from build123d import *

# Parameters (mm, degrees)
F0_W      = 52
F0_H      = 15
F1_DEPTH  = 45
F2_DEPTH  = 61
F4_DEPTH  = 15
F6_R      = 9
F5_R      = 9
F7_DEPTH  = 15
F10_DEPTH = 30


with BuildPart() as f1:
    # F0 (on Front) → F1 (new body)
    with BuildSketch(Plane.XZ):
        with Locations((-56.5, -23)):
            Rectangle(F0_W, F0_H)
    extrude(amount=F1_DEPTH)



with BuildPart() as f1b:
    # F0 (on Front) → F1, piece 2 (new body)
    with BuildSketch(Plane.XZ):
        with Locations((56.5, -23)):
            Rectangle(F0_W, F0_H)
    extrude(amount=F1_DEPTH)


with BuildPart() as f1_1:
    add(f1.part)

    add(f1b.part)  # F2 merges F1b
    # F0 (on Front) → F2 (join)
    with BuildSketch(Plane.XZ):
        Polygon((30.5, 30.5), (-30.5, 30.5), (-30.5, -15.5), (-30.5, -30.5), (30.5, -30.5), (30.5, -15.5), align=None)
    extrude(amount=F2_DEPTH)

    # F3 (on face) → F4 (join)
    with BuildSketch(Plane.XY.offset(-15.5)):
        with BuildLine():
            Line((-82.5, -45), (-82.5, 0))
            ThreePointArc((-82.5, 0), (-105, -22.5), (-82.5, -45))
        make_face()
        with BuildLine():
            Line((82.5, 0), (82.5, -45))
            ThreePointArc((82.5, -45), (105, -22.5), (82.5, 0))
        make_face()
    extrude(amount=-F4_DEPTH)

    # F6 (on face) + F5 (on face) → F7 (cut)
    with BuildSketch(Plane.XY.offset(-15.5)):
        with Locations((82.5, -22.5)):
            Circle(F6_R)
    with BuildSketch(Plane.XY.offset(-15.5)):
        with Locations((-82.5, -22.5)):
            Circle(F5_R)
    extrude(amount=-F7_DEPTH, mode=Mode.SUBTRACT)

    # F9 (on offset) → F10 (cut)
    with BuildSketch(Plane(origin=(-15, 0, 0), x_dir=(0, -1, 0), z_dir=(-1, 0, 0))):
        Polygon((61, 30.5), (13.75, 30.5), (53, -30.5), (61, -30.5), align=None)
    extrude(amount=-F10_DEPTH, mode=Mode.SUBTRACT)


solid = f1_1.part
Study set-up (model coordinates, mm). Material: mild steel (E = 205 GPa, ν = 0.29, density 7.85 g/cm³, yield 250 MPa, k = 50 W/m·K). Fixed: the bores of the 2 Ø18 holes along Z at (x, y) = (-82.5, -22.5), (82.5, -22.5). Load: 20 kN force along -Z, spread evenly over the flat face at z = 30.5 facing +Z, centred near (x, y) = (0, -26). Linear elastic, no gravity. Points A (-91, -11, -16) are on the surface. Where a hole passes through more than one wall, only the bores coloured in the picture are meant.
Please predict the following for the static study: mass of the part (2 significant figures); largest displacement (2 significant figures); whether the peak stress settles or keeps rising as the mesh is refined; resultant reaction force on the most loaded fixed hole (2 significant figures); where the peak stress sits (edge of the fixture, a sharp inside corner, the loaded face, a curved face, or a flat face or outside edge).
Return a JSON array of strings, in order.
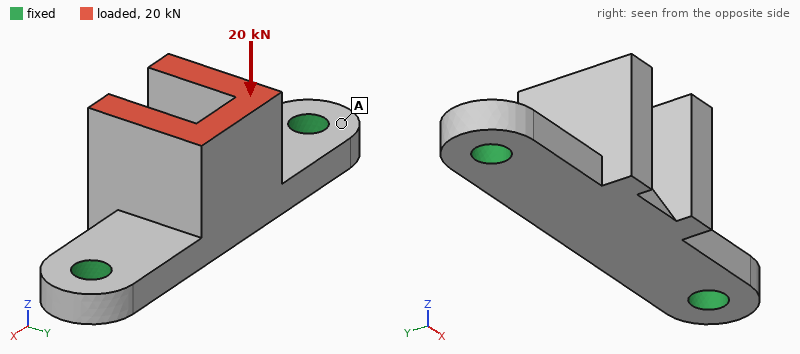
["2.1 kg", "89 µm", "keeps rising", "11 kN", "edge of the fixture"]
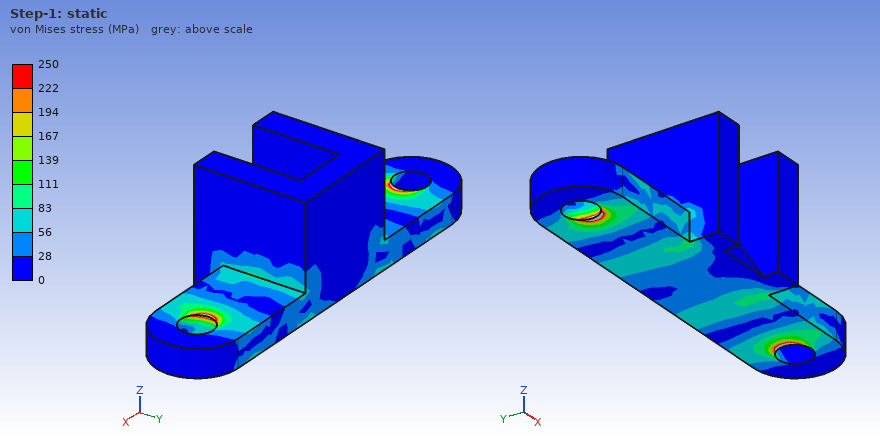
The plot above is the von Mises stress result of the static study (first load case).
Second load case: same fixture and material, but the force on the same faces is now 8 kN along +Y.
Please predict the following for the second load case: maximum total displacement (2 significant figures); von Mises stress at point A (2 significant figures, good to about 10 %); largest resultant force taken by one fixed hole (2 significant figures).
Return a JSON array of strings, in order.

["0.21 mm", "18 MPa", "4.0 kN"]
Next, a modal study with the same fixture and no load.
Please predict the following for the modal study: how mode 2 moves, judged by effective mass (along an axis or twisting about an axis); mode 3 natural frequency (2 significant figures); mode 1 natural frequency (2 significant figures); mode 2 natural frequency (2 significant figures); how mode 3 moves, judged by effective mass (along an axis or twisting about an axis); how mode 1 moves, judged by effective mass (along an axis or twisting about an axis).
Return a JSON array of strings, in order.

["along Z", "3600 Hz", "1500 Hz", "2300 Hz", "along X", "along Y"]
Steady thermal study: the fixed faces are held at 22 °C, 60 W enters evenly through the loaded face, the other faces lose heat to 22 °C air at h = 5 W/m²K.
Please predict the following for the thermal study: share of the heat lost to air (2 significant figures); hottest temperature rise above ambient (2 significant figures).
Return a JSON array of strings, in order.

["11 %", "67 K"]
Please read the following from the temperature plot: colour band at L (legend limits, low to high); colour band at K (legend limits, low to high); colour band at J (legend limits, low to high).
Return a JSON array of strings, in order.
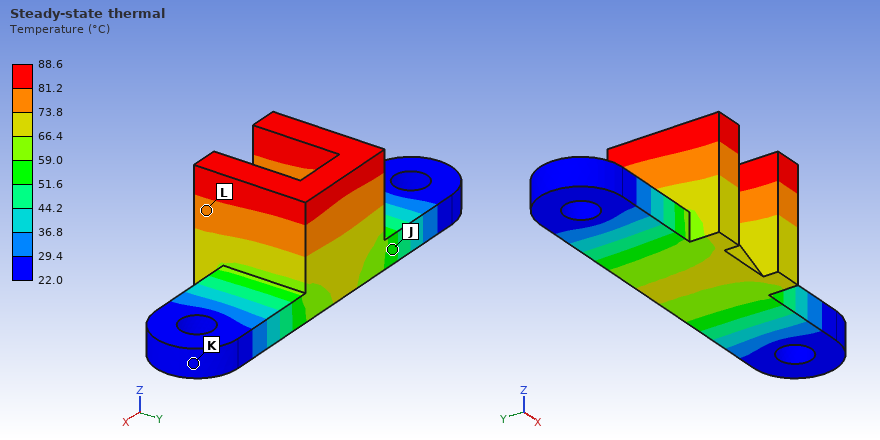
["73.8 to 81.2 °C", "22.0 to 29.4 °C", "51.6 to 59.0 °C"]
